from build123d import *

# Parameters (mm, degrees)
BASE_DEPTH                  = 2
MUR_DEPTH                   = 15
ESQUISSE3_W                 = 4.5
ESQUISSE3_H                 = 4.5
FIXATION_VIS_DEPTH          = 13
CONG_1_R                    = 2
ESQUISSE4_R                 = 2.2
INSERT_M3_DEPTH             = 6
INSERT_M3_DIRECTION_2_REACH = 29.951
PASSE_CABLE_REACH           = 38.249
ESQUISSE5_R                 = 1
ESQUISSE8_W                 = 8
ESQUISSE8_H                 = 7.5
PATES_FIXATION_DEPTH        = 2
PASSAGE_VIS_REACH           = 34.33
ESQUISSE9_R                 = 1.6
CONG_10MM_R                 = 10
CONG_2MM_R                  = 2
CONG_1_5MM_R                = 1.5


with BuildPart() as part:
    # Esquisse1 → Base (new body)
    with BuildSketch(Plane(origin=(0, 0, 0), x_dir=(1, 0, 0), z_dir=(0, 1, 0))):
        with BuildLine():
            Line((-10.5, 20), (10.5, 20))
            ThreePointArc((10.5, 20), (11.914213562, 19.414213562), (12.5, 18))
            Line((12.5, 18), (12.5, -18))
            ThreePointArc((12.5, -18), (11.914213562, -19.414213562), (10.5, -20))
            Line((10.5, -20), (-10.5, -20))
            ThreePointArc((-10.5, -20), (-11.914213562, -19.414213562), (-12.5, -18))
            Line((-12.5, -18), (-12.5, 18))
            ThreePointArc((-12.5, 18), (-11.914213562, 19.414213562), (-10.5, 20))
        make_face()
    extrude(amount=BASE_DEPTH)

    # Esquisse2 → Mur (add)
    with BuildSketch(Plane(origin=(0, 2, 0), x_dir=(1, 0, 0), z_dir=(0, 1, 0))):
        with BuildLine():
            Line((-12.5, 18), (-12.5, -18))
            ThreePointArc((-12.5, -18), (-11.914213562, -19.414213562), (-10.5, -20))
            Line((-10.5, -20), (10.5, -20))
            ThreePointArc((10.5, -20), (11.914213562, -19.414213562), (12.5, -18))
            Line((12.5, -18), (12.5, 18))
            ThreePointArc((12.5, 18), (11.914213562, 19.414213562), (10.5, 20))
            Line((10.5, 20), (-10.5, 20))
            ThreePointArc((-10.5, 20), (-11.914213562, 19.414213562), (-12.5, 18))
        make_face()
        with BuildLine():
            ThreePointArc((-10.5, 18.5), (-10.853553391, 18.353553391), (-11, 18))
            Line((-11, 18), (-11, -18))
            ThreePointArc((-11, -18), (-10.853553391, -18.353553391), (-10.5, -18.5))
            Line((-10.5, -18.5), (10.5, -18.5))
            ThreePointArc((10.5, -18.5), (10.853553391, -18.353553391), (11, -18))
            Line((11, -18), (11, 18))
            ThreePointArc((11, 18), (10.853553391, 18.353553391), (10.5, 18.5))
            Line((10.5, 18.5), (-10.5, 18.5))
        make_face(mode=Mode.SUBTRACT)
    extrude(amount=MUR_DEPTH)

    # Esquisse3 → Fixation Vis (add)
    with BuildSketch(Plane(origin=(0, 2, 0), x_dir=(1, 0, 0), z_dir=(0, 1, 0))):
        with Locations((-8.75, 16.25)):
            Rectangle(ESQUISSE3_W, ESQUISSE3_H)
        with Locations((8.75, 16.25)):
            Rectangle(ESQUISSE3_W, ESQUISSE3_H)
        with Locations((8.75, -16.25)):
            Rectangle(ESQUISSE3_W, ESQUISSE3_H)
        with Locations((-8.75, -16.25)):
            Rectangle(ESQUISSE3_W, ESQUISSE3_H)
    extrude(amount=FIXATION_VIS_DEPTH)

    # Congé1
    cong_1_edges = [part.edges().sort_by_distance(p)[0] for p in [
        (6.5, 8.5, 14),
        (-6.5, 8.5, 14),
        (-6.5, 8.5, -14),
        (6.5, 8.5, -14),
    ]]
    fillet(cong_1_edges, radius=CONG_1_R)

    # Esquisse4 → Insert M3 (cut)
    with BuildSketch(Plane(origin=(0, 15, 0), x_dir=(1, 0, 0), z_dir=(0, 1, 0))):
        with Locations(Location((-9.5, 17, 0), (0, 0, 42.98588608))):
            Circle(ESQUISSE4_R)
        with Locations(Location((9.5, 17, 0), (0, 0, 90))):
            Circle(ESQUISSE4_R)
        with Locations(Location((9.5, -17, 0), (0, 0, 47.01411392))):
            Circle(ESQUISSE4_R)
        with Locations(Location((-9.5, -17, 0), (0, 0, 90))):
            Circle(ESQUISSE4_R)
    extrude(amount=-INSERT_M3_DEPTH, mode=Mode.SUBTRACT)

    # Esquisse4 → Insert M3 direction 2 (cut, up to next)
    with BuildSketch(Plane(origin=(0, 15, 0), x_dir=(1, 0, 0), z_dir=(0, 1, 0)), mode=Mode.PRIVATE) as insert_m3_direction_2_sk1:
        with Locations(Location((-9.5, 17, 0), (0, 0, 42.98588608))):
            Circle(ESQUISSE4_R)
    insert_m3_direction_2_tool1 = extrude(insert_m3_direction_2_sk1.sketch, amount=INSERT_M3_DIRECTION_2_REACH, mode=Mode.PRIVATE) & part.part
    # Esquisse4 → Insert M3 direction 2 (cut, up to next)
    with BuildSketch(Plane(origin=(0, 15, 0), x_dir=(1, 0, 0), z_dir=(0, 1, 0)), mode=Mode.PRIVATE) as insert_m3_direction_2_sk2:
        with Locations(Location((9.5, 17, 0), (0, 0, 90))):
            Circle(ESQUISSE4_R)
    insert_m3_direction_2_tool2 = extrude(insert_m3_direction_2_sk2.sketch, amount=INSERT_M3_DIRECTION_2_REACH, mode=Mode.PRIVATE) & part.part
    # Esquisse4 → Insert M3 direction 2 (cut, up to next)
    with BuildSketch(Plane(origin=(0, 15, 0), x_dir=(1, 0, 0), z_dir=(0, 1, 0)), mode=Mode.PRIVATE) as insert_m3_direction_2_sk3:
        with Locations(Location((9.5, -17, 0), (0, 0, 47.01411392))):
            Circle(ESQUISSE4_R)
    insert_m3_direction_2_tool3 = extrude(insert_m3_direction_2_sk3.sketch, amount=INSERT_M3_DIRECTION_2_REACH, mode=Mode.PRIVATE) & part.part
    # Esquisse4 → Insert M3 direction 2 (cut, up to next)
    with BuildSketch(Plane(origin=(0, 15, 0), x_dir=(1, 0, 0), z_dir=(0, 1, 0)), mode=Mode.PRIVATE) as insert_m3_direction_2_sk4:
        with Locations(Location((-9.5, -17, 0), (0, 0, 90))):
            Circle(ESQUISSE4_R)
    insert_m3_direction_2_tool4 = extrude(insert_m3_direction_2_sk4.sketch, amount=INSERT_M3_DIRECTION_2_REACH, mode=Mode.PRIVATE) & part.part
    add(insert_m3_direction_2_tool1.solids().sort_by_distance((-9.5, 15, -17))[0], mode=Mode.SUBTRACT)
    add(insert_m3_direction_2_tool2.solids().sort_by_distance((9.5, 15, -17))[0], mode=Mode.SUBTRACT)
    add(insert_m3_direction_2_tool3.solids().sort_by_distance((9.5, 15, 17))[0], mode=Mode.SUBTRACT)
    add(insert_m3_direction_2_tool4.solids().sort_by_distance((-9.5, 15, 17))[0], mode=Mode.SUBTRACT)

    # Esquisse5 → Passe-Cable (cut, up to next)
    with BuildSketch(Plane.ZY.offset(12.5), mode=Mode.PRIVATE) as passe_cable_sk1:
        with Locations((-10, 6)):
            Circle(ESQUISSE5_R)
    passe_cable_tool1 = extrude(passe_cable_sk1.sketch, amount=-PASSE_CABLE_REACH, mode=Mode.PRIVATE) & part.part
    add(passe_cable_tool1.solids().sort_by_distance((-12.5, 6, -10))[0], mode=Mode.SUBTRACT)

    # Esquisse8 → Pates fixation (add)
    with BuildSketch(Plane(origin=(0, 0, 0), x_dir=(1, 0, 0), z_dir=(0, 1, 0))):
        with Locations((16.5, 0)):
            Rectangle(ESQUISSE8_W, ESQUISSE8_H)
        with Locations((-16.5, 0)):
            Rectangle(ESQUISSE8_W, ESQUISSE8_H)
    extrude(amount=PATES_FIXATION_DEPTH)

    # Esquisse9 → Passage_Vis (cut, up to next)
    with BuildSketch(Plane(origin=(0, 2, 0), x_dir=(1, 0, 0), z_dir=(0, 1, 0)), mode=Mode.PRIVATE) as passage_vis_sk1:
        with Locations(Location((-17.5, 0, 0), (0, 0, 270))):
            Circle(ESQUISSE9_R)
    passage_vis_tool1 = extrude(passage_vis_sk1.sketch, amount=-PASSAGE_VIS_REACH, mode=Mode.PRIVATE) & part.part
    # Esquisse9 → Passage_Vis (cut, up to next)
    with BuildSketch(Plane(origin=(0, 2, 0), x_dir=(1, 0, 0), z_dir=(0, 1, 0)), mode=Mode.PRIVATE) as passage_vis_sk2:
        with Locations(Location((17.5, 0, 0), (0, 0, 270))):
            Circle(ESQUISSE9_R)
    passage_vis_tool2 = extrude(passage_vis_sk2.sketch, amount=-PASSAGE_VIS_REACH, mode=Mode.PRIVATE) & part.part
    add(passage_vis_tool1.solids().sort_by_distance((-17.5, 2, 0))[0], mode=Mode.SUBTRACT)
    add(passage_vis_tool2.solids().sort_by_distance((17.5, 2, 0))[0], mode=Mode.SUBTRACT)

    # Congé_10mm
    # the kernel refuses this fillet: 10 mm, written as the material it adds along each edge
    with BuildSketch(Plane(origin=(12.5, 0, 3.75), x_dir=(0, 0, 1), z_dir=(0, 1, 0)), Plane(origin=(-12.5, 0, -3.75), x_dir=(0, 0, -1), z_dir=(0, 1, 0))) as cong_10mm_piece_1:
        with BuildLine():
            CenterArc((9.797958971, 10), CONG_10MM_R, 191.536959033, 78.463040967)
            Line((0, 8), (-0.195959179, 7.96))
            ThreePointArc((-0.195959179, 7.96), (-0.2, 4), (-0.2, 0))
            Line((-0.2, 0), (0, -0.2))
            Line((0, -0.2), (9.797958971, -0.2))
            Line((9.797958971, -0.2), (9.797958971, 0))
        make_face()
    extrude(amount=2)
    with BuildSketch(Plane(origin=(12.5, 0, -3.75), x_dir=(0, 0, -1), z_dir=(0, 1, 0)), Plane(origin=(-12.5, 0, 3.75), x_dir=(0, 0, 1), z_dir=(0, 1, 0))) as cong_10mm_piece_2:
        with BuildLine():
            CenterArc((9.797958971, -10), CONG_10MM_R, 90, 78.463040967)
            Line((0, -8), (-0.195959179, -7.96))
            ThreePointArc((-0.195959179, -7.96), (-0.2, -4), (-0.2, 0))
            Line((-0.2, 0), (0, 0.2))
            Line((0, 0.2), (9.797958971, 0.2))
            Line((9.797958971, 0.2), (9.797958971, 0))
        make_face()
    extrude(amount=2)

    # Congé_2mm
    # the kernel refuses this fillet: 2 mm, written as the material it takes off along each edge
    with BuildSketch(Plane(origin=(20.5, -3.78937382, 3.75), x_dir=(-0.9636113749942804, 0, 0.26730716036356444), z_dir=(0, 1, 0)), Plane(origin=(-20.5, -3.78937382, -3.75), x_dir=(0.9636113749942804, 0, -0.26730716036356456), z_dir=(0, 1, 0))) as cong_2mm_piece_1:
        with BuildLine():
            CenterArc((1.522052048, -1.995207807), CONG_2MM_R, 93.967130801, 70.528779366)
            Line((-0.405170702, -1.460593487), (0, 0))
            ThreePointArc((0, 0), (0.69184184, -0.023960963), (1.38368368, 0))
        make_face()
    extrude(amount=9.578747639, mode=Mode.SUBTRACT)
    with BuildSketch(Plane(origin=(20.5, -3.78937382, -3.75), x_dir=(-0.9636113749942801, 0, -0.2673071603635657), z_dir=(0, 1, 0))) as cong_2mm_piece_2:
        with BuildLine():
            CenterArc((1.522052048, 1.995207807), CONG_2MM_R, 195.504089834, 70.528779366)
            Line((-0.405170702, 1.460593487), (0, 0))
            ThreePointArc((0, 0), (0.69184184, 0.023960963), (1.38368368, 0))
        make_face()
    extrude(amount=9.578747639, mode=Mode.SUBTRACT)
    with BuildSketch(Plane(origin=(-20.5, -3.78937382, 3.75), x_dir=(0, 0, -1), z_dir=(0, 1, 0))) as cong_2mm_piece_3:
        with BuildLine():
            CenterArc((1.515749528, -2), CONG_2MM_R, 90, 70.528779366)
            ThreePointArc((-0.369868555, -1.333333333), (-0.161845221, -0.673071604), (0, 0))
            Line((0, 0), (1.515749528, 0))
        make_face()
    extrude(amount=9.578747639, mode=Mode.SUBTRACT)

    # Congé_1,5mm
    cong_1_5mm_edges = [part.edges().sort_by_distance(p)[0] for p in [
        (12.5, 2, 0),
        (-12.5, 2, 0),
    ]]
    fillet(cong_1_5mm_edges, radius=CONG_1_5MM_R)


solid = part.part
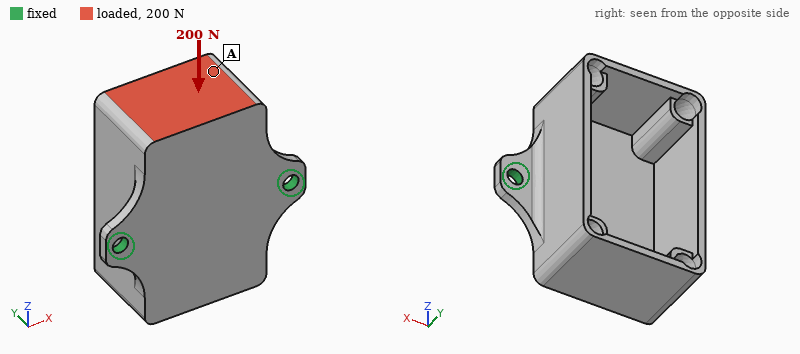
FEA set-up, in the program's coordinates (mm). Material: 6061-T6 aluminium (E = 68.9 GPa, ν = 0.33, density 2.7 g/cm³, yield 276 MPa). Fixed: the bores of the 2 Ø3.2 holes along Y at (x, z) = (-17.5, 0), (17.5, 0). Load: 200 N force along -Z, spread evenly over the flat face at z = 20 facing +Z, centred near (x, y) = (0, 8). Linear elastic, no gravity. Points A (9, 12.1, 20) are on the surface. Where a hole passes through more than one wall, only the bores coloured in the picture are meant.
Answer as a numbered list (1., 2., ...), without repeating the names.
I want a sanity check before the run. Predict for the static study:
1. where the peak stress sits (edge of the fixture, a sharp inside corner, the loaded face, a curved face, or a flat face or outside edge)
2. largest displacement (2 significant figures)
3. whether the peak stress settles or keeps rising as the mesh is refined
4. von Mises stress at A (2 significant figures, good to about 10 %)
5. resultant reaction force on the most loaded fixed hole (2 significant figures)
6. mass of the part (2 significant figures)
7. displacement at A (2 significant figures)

1. edge of the fixture
2. 88 µm
3. keeps rising
4. 12 MPa
5. 100 N
6. 15 g
7. 70 µm
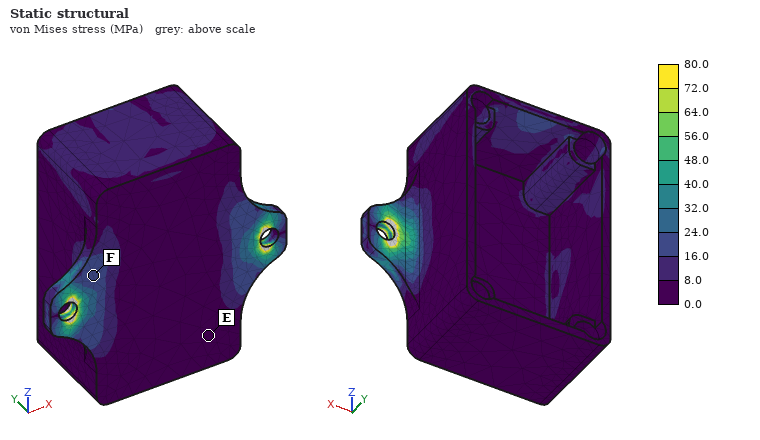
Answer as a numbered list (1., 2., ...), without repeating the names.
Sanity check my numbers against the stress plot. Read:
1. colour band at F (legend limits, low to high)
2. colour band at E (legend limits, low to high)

1. 16.0 to 24.0 MPa
2. 0.0 to 8.0 MPa
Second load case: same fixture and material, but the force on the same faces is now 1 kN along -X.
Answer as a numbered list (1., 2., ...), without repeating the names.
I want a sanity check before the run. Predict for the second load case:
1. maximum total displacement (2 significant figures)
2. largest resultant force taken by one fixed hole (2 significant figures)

1. 0.16 mm
2. 800 N
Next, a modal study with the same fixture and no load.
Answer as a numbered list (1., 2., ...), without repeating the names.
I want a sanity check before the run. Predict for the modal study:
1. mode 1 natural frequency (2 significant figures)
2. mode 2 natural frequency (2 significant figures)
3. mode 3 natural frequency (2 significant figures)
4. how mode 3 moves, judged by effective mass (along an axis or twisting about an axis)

1. 2000 Hz
2. 5000 Hz
3. 6600 Hz
4. along Y
